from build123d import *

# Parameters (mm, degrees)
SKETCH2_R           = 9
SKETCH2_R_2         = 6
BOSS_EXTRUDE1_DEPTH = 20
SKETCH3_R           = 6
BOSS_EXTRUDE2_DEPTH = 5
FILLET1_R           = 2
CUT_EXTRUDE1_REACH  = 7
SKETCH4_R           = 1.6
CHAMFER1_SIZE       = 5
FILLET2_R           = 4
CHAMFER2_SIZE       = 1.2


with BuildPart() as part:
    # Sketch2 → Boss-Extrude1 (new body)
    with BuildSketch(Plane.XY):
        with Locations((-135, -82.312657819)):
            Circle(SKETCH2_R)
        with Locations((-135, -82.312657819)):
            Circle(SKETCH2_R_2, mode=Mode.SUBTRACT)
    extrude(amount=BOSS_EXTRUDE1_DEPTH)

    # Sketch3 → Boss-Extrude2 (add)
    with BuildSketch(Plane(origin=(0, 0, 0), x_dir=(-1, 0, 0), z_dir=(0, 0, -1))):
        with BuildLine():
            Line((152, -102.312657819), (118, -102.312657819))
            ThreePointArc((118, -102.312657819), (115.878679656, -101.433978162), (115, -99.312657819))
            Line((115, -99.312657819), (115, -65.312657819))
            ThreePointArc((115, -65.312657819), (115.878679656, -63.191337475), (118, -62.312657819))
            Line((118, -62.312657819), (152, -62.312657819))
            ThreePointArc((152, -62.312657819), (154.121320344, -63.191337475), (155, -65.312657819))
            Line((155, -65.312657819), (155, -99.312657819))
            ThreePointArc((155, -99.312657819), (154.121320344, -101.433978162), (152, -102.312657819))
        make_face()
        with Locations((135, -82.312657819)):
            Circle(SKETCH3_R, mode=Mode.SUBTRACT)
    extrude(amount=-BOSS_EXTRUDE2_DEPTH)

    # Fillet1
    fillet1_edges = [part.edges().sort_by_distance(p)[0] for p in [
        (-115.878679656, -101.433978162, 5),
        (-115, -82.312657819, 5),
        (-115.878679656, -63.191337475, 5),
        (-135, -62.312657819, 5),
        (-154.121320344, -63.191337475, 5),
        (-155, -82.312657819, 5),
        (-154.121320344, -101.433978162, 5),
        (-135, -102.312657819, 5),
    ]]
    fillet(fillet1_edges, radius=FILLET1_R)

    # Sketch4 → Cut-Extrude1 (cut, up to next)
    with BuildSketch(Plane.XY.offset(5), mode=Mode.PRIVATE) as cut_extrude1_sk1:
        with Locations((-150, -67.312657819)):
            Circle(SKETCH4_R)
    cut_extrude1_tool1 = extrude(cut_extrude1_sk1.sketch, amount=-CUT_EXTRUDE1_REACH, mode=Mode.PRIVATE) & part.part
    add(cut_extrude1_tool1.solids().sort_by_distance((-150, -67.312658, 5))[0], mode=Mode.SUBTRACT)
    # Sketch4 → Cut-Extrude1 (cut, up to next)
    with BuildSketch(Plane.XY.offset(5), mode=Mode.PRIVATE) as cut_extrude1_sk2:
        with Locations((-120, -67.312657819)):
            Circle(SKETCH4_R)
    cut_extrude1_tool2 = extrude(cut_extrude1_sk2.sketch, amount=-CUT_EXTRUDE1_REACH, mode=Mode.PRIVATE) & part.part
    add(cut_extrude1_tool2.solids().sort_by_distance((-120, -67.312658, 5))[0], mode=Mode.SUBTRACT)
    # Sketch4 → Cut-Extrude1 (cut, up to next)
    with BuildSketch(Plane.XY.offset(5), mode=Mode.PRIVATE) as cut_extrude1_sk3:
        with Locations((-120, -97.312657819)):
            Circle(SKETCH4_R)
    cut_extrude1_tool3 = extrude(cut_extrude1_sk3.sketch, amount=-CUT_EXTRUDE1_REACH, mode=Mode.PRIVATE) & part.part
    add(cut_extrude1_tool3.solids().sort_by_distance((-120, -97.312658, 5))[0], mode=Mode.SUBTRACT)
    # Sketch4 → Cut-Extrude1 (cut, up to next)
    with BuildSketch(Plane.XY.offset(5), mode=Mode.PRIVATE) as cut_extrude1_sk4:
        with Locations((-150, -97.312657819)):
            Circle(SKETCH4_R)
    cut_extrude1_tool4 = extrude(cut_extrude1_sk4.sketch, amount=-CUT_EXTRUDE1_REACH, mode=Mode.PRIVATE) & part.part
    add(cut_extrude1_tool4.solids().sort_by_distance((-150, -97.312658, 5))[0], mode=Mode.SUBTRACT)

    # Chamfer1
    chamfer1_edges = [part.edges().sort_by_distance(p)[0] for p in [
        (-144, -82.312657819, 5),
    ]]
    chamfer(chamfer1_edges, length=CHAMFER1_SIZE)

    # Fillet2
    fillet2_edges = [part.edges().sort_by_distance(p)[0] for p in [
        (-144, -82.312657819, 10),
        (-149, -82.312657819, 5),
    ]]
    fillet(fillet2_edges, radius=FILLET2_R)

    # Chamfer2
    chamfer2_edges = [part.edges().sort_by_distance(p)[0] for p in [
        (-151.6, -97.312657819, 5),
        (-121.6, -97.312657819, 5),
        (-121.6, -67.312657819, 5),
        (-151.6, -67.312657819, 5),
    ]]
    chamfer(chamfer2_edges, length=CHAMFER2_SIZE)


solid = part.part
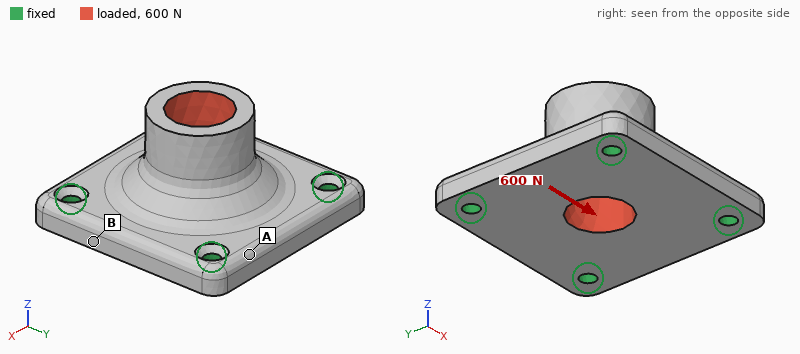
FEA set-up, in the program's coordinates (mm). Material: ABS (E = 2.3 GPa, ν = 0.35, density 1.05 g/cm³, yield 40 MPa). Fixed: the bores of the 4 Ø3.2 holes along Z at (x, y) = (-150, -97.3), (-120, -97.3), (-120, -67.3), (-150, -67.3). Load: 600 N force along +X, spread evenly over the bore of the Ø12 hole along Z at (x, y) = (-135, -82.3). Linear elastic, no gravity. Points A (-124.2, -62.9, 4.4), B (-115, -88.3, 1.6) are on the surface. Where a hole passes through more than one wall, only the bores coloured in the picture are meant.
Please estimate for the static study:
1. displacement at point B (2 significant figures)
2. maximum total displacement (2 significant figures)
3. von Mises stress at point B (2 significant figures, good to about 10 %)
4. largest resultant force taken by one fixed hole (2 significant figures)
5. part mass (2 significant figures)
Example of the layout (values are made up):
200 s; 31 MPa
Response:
0.040 mm; 0.12 mm; 2.7 MPa; 190 N; 11 g
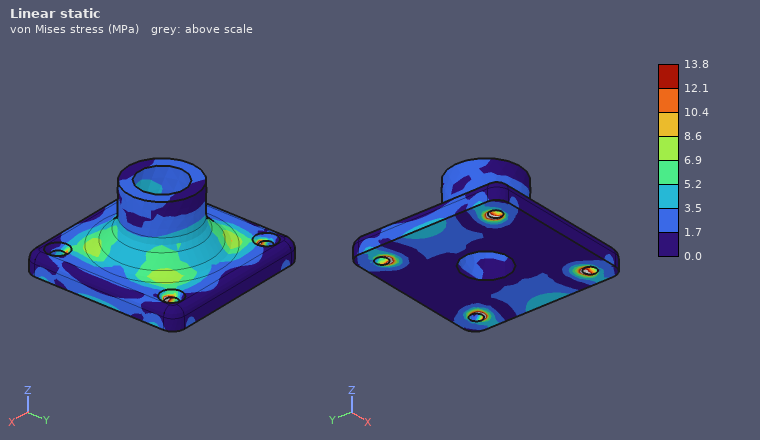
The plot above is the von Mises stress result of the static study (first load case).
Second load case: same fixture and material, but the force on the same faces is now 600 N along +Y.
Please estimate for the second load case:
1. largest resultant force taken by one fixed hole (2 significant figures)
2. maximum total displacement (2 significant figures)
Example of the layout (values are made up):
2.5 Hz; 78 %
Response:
190 N; 0.12 mm
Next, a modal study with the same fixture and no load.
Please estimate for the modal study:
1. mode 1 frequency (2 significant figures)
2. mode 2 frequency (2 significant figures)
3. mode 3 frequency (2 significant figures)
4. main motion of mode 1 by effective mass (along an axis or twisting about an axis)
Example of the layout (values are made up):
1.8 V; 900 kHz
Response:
5000 Hz; 6000 Hz; 6000 Hz; along Z
